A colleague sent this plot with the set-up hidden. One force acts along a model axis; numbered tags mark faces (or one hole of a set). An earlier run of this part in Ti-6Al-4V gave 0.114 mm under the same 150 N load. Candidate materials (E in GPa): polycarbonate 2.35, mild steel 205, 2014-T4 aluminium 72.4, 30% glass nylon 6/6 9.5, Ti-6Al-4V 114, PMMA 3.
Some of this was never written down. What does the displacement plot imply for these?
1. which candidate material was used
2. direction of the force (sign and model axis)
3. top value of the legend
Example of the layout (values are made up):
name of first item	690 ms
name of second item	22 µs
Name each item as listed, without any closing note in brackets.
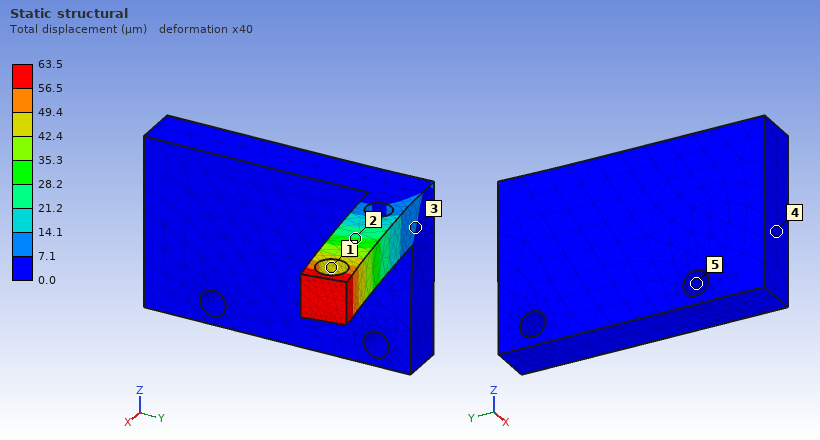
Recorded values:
which candidate material was used	mild steel
direction of the force	+Y
top value of the legend	63.5 µm
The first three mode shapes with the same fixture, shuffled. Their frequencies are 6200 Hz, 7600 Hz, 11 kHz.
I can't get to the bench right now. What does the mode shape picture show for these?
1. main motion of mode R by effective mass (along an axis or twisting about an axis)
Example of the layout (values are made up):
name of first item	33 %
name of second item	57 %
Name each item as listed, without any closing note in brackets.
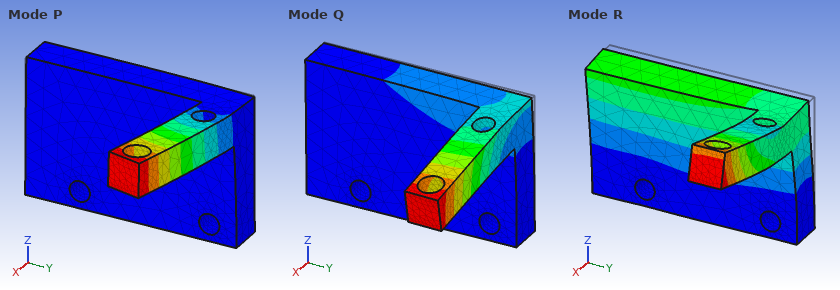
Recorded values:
main motion of mode R by effective mass	along X
